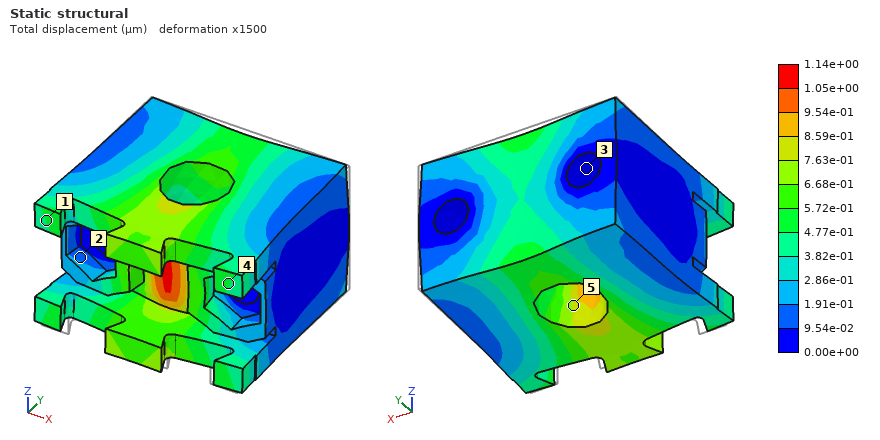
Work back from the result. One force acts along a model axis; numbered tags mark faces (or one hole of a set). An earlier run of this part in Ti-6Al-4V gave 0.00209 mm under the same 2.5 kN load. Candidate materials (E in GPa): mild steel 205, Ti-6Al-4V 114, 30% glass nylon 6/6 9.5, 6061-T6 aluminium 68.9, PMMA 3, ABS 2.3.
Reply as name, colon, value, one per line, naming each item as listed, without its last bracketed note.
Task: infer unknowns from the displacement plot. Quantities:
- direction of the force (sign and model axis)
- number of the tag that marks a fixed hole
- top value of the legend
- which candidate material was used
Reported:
direction of the force: -Y
number of the tag that marks a fixed hole: 3
top value of the legend: 1.14e+00 µm
which candidate material was used: mild steel
